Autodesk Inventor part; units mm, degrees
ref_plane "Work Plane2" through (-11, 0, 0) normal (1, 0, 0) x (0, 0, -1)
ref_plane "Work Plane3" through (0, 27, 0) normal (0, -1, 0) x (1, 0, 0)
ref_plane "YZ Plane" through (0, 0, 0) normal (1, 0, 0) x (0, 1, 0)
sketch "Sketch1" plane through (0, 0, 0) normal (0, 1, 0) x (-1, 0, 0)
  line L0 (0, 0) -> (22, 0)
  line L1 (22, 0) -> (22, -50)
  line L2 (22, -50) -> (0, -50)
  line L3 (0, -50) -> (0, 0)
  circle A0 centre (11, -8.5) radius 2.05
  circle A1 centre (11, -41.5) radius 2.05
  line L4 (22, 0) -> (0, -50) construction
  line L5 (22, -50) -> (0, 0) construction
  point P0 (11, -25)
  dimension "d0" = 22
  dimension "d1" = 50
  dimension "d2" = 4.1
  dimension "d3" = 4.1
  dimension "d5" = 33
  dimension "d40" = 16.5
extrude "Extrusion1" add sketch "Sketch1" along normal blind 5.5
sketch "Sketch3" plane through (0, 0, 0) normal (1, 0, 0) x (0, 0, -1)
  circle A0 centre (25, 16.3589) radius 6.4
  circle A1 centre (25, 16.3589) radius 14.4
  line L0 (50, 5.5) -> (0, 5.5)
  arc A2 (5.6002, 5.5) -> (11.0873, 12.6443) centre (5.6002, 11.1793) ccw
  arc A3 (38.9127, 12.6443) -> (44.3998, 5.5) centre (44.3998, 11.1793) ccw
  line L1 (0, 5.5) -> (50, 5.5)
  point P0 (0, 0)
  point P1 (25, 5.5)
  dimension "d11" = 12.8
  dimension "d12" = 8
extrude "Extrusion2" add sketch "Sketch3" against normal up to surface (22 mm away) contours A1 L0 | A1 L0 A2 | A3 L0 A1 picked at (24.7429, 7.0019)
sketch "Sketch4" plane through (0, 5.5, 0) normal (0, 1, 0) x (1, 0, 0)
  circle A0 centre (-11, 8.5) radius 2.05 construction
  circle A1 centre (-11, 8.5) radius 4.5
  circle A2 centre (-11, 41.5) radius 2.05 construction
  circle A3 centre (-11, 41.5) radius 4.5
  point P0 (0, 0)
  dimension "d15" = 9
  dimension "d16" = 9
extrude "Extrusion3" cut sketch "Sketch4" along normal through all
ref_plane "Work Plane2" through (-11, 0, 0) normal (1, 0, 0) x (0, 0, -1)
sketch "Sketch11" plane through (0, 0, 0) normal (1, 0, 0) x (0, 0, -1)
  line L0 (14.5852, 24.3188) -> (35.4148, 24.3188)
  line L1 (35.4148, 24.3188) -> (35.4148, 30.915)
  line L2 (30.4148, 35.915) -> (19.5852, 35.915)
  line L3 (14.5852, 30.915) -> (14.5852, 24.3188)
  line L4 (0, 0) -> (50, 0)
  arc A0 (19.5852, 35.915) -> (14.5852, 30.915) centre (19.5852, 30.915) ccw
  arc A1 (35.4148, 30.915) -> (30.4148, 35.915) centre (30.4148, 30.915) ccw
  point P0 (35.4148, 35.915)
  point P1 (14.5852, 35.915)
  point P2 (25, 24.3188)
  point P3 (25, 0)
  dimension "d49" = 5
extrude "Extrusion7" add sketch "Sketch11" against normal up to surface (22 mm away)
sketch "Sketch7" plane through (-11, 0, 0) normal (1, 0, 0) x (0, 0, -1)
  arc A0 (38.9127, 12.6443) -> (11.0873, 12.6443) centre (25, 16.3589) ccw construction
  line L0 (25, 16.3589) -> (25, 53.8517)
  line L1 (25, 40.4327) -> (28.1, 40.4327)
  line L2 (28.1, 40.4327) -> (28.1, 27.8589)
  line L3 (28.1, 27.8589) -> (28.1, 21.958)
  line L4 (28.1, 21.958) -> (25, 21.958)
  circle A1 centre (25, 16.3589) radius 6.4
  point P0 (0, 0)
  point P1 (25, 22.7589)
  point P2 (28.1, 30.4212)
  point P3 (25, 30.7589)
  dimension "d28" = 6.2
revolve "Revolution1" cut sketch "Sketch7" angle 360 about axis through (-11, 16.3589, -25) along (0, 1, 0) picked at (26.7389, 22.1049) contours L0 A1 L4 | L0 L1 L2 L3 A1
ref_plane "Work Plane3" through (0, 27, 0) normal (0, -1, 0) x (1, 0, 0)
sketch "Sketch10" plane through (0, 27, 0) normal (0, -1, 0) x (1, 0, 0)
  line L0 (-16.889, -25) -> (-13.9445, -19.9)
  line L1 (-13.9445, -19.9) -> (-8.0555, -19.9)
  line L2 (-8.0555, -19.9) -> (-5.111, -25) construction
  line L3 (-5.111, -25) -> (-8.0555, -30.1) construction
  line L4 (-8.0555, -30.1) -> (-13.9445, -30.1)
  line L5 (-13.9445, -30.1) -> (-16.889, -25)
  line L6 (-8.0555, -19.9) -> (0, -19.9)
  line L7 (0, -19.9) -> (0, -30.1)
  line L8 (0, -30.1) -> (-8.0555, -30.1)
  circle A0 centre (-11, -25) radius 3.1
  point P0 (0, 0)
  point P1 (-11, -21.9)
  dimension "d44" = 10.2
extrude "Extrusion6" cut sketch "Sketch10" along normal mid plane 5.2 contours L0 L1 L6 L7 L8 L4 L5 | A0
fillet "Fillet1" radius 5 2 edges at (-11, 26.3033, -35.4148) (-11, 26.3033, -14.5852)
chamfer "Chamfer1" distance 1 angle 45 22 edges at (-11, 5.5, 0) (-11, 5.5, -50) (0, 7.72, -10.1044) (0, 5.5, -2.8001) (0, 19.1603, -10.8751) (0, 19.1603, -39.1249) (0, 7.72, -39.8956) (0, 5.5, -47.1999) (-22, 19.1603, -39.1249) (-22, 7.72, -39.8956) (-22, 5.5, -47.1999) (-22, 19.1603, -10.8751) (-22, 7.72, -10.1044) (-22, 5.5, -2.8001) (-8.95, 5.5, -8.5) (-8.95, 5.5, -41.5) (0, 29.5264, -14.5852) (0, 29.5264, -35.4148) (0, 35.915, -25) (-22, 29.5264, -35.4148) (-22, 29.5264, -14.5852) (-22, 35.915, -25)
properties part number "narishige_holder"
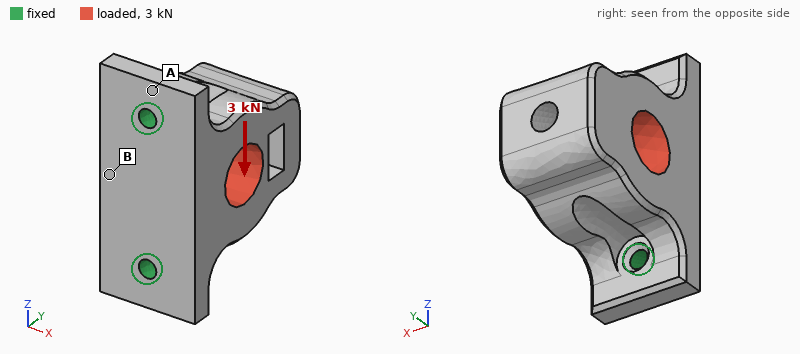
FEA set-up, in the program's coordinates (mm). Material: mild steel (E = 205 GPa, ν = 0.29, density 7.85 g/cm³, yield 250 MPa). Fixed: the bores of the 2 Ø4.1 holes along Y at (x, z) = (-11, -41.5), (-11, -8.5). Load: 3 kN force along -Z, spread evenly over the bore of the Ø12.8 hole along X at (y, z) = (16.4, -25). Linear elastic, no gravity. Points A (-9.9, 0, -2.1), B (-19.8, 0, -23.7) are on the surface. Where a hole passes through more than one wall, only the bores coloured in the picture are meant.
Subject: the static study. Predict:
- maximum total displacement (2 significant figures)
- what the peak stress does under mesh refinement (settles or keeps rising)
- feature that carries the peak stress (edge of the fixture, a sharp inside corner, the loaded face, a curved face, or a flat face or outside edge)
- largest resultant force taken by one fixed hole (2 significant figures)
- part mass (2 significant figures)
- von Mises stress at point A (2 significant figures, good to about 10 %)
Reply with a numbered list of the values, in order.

1. 6.6 µm
2. keeps rising
3. edge of the fixture
4. 2.0 kN
5. 140 g
6. 19 MPa
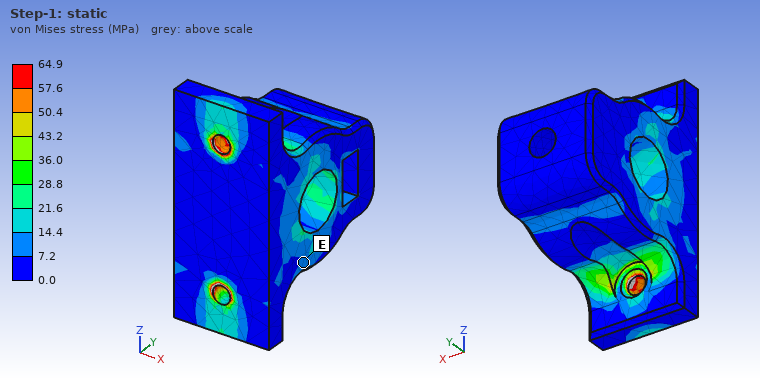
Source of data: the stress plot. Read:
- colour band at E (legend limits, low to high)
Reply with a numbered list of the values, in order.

1. 7.2 to 14.4 MPa
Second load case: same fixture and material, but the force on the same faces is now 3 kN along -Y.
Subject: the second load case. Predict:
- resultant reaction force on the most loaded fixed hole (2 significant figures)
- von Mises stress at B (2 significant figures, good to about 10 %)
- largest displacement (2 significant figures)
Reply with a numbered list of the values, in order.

1. 1.7 kN
2. 9.2 MPa
3. 3.1 µm
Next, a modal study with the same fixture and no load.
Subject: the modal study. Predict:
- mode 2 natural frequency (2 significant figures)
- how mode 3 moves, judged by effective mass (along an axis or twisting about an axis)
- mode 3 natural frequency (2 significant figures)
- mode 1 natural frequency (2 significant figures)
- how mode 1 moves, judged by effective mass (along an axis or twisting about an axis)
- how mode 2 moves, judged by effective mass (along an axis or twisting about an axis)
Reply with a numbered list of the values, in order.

1. 11 kHz
2. along Y
3. 16 kHz
4. 4000 Hz
5. along X
6. along Z
